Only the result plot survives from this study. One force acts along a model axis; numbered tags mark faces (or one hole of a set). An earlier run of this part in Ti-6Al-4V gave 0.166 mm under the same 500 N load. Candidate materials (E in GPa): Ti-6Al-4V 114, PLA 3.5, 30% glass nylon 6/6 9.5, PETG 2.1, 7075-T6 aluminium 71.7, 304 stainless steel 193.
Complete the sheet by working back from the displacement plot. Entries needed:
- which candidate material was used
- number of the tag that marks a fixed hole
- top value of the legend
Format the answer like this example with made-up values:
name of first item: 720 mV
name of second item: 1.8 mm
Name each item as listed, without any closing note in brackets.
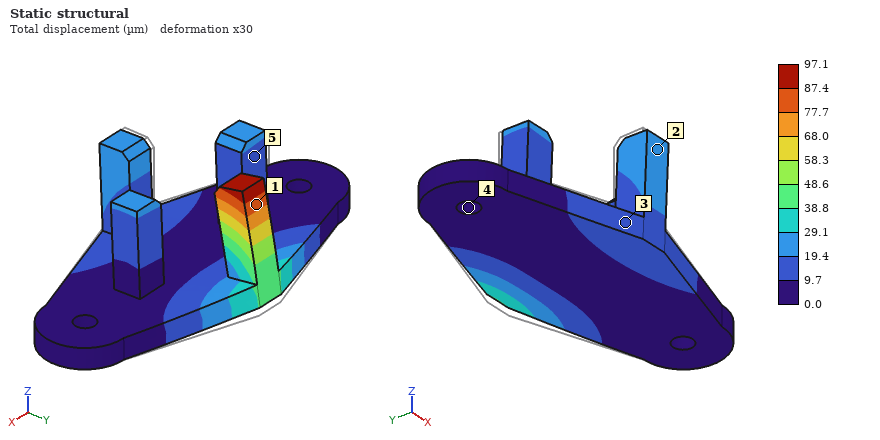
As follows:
which candidate material was used: 304 stainless steel
number of the tag that marks a fixed hole: 4
top value of the legend: 97.1 µm
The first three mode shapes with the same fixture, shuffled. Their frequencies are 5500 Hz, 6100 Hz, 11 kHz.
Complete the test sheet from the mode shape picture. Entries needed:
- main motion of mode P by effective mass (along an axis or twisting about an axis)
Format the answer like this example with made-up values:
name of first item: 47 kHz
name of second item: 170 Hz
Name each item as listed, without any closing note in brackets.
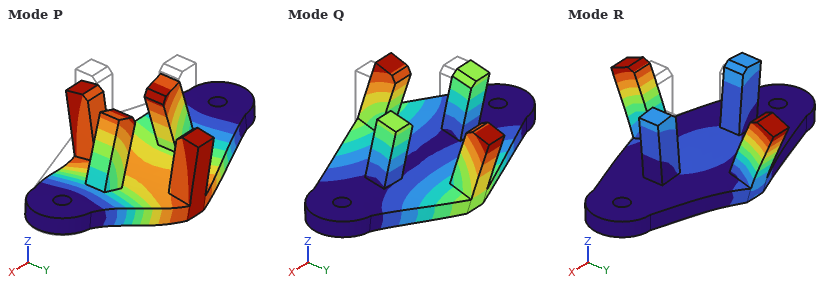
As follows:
main motion of mode P by effective mass: along Z
